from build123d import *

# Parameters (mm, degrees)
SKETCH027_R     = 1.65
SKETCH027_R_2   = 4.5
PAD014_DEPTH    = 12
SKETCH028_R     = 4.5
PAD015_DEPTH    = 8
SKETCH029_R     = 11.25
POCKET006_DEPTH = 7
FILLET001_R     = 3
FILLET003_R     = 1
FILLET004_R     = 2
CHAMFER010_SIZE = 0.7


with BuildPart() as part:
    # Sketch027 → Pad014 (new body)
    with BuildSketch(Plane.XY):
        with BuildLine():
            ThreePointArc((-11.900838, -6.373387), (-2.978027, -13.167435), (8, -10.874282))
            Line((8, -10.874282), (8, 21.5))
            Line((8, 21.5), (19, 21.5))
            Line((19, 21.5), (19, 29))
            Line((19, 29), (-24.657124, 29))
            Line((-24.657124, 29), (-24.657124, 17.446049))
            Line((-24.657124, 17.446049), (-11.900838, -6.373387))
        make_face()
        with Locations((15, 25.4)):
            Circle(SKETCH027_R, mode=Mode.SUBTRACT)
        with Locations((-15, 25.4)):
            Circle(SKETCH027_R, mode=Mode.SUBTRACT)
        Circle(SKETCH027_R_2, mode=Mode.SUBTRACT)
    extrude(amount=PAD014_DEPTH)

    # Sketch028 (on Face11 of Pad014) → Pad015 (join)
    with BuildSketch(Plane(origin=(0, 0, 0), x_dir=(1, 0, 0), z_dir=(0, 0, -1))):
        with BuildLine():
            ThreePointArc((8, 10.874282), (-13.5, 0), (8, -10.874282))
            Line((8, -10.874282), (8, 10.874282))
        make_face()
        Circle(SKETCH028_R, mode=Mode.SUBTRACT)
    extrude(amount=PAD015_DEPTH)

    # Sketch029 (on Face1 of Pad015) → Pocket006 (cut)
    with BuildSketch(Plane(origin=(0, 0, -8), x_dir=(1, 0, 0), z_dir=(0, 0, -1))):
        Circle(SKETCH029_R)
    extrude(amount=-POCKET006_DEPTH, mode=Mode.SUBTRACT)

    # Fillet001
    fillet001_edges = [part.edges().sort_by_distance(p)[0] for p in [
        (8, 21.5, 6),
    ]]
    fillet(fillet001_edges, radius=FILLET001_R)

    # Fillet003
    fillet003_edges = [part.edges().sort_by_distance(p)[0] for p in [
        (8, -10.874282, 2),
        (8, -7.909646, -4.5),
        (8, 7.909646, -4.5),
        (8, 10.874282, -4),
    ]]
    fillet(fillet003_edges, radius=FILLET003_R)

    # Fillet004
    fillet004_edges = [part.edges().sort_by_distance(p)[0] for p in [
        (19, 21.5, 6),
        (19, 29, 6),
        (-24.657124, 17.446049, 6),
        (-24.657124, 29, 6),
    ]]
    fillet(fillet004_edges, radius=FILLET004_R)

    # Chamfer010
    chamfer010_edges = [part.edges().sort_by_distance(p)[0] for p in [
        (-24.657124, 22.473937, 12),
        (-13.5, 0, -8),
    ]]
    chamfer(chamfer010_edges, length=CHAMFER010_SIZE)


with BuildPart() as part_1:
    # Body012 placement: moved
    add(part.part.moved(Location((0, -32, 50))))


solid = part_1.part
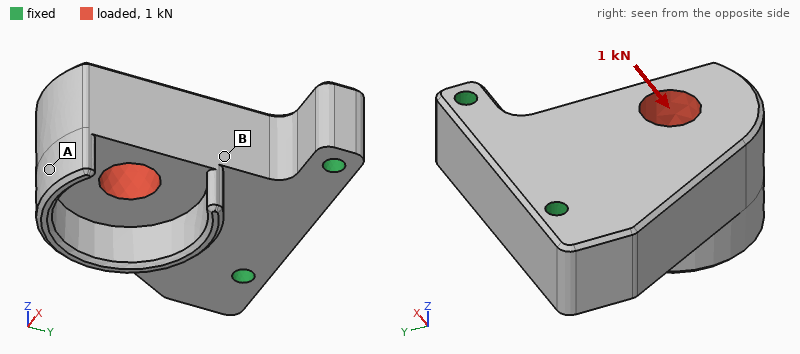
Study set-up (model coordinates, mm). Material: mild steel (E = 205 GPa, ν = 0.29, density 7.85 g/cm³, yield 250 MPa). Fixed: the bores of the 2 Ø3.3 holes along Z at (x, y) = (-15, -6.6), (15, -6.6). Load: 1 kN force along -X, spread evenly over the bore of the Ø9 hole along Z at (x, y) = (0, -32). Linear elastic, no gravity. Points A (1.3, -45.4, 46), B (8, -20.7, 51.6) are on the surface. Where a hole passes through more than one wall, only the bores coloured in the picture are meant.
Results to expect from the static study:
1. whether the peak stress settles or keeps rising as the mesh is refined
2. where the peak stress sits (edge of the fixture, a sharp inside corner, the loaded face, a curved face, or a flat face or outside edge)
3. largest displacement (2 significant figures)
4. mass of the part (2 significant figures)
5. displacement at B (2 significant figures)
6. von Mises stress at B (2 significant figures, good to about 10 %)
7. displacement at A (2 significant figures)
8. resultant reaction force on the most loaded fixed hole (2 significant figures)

keeps rising
edge of the fixture
5.5 µm
110 g
2.6 µm
8.3 MPa
5.5 µm
1.0 kN
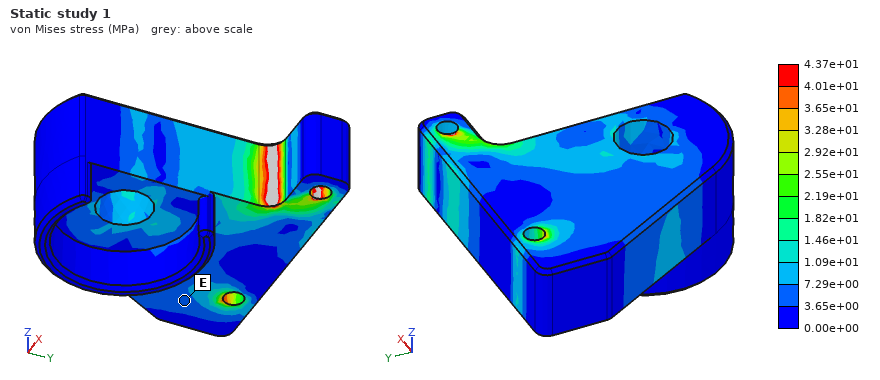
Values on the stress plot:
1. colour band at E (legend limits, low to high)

3.65e+00 to 7.29e+00 MPa
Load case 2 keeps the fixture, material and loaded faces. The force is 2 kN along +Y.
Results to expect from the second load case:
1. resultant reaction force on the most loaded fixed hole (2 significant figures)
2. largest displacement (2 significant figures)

1.1 kN
5.8 µm
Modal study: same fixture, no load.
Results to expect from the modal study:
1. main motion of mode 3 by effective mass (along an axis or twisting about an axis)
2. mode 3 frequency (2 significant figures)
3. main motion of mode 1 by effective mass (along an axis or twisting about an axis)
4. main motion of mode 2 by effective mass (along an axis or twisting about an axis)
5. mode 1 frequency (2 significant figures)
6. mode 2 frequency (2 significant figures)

twisting about Y
17 kHz
along Z
along X
5300 Hz
10 kHz
